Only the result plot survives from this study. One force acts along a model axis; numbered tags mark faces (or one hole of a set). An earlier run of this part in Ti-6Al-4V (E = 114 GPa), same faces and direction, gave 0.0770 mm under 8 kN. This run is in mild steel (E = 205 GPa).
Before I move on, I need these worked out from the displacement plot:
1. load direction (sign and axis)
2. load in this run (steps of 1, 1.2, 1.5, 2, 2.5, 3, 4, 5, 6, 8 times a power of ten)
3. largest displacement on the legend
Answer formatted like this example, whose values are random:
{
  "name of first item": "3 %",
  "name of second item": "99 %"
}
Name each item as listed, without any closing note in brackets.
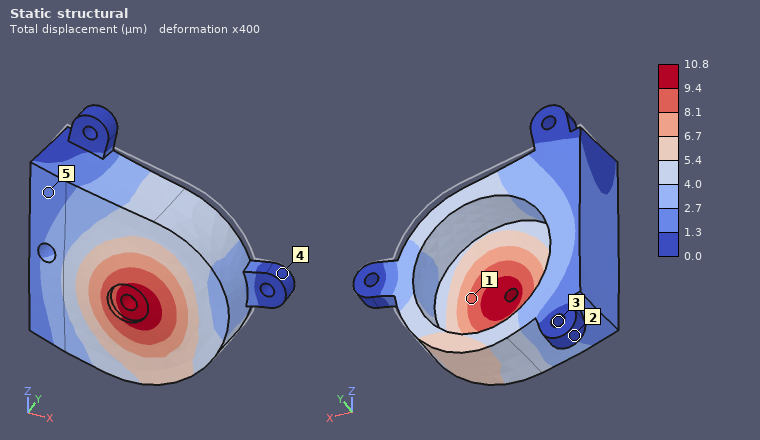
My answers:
{
  "load direction": "-Y",
  "load in this run": "2 kN",
  "largest displacement on the legend": "10.8 µm"
}
